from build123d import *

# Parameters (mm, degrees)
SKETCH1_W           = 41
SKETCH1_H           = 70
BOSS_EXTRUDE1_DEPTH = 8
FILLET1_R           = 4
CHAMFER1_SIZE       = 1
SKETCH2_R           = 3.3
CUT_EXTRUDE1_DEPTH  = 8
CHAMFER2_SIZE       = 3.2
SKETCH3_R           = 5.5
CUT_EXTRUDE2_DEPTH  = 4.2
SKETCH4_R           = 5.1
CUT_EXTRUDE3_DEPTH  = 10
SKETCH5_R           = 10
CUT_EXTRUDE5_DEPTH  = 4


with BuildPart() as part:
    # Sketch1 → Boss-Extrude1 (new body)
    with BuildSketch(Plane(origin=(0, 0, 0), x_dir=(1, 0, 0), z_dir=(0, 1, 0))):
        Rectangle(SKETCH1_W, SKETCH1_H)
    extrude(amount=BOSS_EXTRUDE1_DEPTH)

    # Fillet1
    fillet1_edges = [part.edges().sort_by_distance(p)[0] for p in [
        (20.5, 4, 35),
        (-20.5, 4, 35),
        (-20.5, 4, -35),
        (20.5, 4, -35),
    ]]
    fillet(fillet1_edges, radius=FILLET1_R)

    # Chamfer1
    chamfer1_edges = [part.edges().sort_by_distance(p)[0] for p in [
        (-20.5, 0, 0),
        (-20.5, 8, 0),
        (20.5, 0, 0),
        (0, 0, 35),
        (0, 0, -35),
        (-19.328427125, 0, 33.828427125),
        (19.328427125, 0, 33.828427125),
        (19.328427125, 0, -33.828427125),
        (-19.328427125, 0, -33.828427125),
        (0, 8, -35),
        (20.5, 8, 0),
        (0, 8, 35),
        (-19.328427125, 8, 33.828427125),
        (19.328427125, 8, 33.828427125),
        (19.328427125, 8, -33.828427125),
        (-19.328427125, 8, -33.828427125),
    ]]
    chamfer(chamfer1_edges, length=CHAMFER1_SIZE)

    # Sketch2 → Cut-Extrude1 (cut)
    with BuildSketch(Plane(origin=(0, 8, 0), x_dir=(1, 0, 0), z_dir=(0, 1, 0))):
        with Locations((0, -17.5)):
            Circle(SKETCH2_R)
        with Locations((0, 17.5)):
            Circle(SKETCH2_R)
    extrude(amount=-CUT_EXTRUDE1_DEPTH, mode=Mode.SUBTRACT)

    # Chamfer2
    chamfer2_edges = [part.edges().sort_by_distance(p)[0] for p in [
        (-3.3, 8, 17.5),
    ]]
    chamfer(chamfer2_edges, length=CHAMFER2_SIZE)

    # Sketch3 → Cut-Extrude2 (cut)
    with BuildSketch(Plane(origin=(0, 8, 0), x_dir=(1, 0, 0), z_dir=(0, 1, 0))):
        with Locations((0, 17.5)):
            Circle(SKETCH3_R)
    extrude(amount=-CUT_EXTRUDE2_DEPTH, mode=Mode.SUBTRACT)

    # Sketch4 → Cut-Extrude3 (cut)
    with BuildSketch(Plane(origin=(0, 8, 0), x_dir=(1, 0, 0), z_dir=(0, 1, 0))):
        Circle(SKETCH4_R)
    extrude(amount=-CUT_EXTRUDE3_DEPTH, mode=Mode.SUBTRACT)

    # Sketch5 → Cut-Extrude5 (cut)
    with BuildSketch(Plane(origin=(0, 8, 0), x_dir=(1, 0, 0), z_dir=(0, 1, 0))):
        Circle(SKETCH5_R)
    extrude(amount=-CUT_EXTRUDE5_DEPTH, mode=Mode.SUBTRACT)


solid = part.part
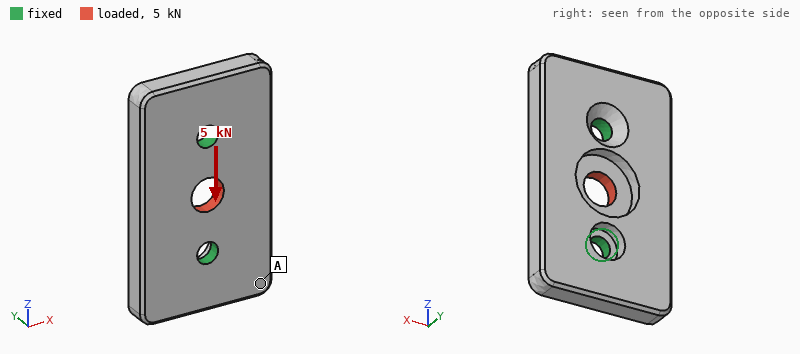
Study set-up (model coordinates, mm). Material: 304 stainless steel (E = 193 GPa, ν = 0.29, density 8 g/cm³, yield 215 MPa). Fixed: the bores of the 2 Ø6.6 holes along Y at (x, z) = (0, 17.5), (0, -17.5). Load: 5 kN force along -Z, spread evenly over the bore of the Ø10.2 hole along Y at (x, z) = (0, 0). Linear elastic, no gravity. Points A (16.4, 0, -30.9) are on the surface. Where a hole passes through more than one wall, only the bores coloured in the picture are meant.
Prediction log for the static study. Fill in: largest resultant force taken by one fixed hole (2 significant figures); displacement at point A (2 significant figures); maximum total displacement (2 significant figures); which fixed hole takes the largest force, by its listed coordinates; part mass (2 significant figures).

2.7 kN
0.92 µm
2.6 µm
(0, 17.5)
160 g
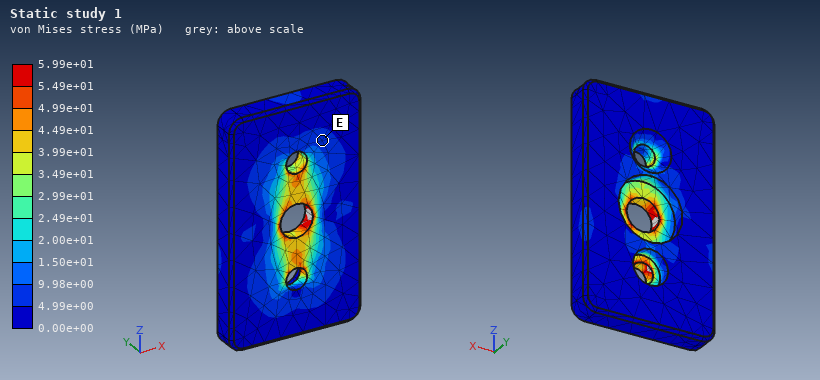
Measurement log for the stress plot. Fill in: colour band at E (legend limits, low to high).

4.99e+00 to 9.98e+00 MPa
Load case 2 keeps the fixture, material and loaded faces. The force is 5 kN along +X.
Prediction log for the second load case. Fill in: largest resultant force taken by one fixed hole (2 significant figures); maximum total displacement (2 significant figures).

2.5 kN
4.2 µm
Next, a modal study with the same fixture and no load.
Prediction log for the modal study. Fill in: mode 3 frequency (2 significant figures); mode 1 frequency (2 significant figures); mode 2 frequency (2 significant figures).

11 kHz
6700 Hz
9900 Hz
